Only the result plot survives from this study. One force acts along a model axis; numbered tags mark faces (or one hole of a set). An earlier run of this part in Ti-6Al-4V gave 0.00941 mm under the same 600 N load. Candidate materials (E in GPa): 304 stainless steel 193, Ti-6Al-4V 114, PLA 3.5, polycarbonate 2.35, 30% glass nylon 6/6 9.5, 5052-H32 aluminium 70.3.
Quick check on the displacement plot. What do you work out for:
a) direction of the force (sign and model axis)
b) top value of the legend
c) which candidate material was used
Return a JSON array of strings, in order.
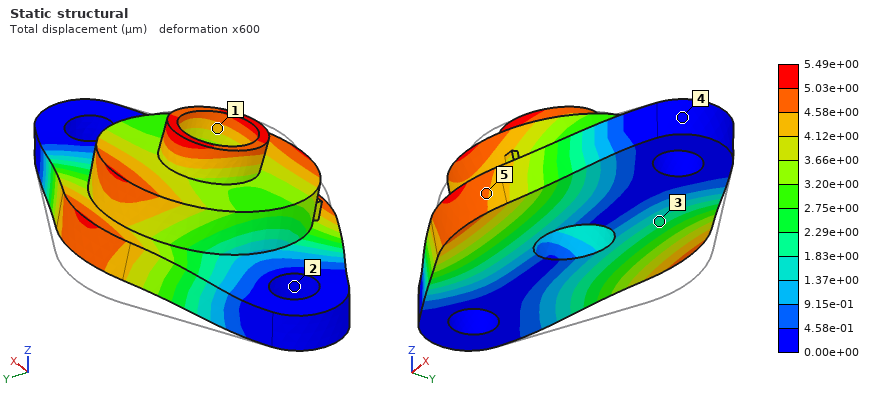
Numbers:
["-Y", "5.49e+00 µm", "304 stainless steel"]
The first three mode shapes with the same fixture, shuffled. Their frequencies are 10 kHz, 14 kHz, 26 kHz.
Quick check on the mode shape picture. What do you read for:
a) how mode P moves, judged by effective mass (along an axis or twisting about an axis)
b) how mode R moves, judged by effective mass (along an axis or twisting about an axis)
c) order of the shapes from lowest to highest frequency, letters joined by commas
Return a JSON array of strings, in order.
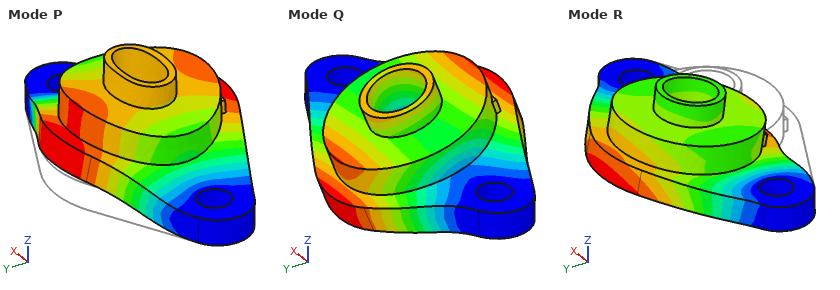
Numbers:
["along Z", "along Y", "Q, P, R"]
